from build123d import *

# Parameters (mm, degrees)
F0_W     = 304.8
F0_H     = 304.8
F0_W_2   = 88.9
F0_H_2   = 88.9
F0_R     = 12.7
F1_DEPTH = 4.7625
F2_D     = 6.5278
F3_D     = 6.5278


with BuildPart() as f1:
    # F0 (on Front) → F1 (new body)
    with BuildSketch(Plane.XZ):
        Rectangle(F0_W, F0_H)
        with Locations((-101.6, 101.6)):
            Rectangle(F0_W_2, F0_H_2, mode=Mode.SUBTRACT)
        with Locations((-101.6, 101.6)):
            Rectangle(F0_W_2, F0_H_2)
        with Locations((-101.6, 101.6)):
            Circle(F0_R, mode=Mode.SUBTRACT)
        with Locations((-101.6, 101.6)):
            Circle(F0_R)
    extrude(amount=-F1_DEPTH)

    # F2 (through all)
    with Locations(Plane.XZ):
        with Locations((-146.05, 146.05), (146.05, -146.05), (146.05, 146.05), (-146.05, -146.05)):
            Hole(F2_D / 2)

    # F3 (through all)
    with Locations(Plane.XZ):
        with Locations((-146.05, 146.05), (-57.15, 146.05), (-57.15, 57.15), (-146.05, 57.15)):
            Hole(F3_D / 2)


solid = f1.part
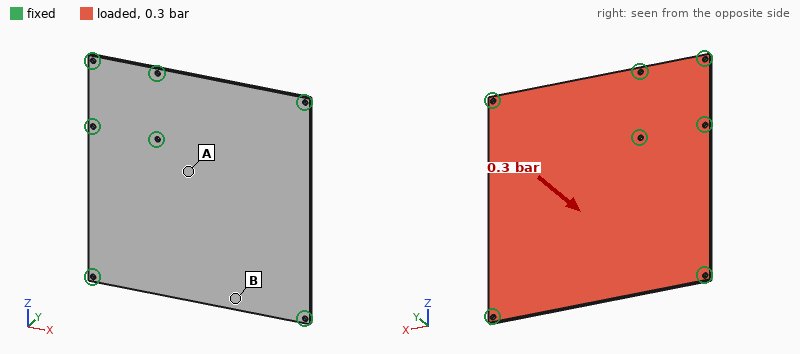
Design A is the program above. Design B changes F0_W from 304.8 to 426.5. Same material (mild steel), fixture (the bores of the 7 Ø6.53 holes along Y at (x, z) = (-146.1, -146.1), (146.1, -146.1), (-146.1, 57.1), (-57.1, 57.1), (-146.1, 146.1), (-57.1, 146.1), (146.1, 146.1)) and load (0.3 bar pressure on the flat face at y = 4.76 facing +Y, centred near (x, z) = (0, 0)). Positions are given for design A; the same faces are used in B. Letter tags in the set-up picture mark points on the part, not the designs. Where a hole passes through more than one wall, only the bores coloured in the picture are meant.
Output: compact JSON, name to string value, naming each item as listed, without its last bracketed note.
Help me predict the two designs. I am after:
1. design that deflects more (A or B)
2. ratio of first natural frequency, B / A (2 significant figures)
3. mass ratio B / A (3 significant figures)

{"design that deflects more": "B", "ratio of first natural frequency, B / A": "0.99", "mass ratio B / A": "1.40"}
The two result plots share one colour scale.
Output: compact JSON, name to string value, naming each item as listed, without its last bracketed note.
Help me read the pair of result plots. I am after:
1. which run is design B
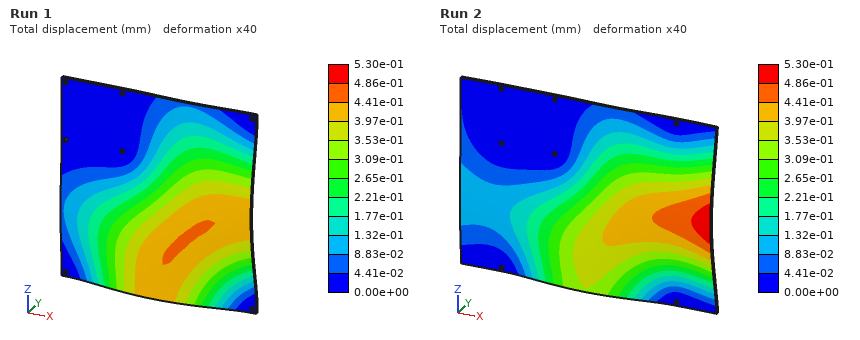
{"which run is design B": "Run 2"}
